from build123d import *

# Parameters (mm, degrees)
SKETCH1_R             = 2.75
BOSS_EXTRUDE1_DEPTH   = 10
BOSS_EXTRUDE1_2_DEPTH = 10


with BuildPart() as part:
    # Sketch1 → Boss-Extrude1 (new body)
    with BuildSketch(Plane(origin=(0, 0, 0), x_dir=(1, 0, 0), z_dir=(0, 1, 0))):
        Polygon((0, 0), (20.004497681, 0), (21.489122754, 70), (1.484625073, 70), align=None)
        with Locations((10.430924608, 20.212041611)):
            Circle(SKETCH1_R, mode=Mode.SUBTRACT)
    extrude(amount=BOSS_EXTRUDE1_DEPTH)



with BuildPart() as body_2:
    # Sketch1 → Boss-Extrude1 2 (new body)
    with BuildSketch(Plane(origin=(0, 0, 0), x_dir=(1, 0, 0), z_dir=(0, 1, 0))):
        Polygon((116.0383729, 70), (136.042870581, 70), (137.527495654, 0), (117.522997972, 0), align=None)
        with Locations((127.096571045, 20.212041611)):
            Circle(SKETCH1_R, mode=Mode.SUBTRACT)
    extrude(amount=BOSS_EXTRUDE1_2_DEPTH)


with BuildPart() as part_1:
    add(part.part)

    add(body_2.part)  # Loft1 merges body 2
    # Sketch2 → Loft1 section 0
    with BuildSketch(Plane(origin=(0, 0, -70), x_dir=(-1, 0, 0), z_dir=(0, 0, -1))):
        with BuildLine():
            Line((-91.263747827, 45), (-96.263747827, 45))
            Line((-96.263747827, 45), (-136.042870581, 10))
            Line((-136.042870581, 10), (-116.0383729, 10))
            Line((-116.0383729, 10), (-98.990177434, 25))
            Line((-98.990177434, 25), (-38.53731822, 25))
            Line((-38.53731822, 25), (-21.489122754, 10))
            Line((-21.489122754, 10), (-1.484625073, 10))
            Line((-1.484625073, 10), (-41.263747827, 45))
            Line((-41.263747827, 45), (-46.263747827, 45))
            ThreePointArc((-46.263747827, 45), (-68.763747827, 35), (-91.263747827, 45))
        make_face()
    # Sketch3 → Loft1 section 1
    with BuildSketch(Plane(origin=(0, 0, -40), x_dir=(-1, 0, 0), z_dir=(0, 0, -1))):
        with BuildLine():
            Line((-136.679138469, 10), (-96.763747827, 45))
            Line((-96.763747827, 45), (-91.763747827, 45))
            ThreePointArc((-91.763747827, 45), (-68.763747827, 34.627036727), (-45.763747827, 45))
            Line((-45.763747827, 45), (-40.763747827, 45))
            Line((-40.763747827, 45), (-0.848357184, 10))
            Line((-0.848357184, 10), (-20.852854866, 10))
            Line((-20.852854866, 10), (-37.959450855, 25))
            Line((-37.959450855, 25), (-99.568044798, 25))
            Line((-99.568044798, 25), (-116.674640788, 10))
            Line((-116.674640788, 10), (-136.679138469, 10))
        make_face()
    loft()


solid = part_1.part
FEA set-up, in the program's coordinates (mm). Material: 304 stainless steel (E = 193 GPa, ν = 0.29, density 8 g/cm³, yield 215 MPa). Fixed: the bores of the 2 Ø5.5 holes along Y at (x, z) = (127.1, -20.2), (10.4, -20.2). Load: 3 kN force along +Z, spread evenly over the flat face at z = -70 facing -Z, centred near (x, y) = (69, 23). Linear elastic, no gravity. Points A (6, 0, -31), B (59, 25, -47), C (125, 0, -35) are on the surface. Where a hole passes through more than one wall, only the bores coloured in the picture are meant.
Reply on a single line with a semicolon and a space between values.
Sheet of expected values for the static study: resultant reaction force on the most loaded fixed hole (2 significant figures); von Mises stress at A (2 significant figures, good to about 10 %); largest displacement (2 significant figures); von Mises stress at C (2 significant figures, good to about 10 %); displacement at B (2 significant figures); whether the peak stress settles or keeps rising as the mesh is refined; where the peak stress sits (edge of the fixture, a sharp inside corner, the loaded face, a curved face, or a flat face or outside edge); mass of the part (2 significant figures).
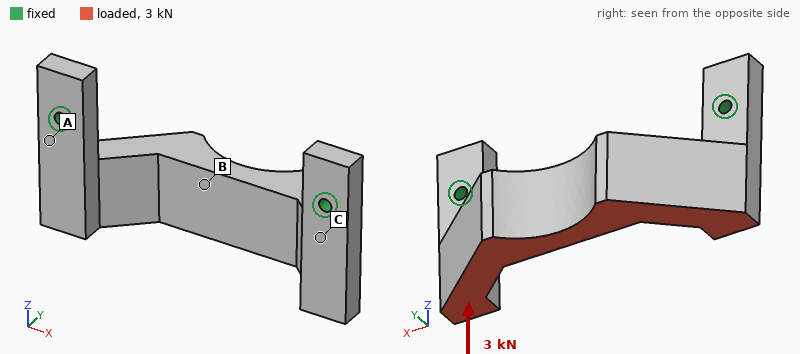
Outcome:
1.5 kN; 79 MPa; 0.13 mm; 70 MPa; 0.064 mm; keeps rising; edge of the fixture; 660 g
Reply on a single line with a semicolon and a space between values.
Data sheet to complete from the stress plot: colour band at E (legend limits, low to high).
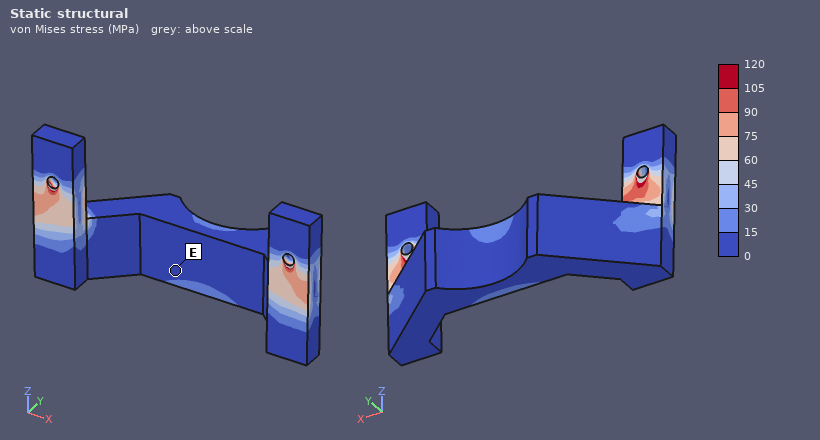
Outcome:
0 to 15 MPa
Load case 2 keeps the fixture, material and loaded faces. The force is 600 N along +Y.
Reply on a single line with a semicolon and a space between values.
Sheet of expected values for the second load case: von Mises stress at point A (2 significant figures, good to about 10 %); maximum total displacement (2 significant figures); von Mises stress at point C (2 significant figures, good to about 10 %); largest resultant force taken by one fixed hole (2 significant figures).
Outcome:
35 MPa; 54 µm; 30 MPa; 320 N
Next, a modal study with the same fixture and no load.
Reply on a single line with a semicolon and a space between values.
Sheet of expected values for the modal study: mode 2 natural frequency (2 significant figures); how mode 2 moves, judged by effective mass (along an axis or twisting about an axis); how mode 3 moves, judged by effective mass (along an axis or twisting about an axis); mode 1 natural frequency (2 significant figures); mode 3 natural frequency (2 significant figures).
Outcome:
2700 Hz; along X; along X; 1000 Hz; 3100 Hz
